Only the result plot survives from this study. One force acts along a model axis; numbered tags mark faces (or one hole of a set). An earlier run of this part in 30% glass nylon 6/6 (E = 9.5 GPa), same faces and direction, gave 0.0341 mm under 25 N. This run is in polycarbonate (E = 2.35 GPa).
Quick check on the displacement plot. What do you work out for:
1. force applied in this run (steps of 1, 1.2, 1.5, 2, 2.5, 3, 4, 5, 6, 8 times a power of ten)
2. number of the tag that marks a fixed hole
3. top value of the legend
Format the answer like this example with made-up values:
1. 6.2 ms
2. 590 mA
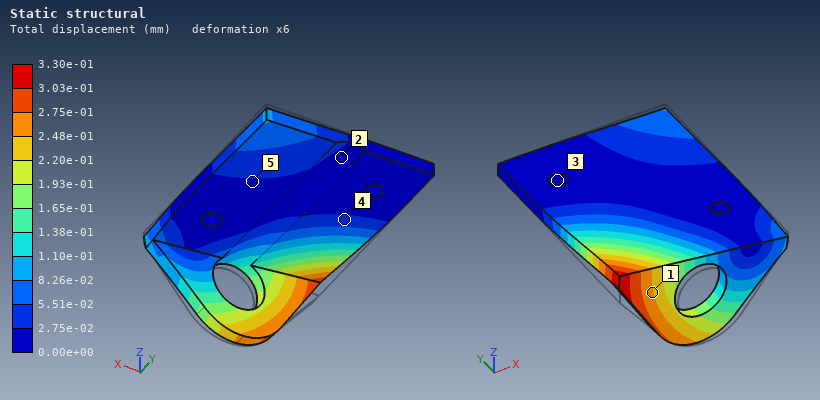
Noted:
1. 60 N
2. 3
3. 3.30e-01 mm
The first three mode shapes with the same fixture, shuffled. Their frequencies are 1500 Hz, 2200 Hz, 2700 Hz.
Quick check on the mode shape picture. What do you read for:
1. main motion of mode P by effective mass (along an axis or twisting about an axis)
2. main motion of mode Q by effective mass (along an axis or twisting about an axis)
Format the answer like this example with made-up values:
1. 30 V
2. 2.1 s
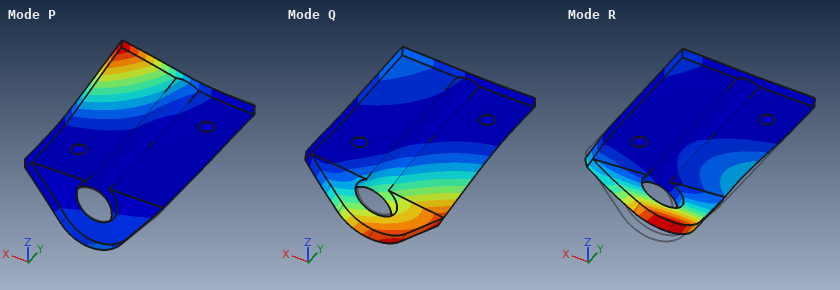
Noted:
1. along Z
2. along Z
